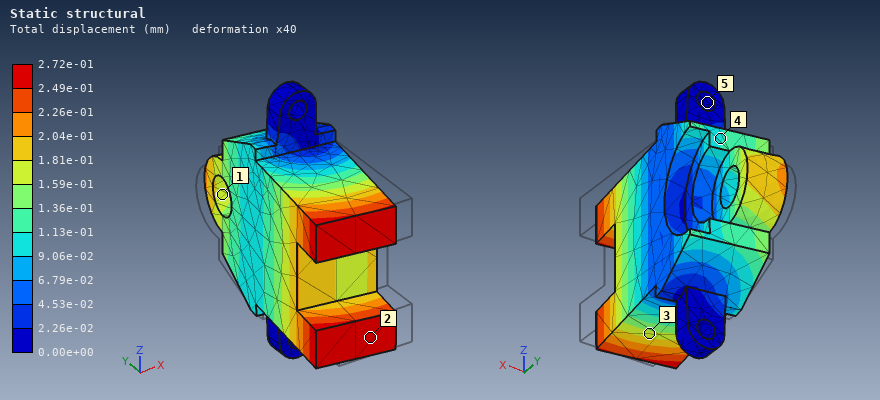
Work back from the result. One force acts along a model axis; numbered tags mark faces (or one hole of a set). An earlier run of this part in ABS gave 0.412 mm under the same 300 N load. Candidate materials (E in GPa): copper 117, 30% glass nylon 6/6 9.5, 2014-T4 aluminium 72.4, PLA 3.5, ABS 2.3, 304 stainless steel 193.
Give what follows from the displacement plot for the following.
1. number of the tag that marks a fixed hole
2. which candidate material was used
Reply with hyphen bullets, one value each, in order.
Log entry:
- 5
- PLA
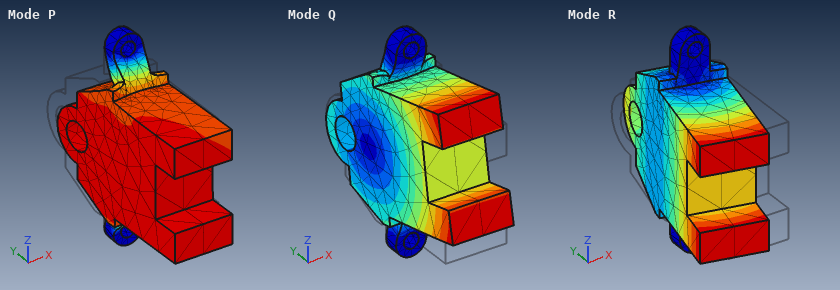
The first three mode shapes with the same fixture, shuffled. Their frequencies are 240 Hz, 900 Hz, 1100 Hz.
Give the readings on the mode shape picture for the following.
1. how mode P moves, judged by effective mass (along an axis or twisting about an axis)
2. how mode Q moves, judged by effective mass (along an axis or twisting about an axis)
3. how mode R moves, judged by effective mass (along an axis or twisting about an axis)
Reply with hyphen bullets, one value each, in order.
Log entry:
- along Y
- along Z
- along X
